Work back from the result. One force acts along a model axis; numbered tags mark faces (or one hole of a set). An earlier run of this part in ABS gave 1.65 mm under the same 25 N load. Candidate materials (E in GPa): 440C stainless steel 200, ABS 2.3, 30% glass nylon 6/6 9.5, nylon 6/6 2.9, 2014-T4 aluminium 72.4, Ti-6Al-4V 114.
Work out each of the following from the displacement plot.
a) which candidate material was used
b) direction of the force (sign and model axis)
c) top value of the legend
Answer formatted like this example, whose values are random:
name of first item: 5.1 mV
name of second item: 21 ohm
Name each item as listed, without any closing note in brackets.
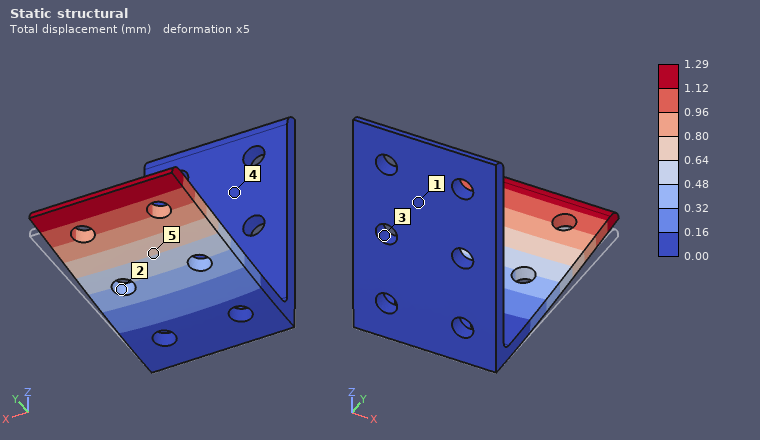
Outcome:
which candidate material was used: nylon 6/6
direction of the force: +Z
top value of the legend: 1.29 mm
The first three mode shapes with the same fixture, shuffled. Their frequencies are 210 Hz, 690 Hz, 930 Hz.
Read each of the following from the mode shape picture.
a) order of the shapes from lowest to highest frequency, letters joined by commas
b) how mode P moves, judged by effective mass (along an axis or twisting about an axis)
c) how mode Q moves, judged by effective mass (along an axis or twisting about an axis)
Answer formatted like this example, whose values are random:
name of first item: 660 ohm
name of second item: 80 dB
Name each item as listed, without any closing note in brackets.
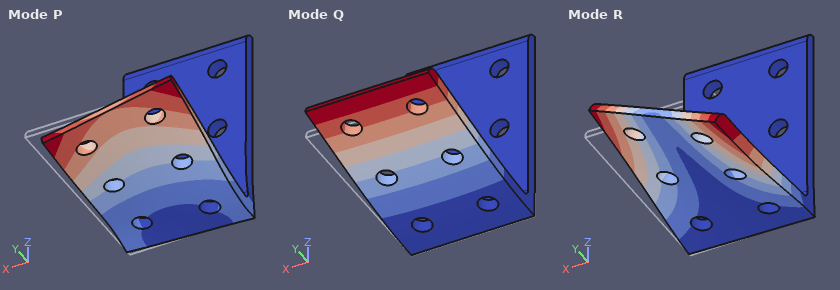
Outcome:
order of the shapes from lowest to highest frequency, letters joined by commas: Q, R, P
how mode P moves, judged by effective mass: along X
how mode Q moves, judged by effective mass: along Z
